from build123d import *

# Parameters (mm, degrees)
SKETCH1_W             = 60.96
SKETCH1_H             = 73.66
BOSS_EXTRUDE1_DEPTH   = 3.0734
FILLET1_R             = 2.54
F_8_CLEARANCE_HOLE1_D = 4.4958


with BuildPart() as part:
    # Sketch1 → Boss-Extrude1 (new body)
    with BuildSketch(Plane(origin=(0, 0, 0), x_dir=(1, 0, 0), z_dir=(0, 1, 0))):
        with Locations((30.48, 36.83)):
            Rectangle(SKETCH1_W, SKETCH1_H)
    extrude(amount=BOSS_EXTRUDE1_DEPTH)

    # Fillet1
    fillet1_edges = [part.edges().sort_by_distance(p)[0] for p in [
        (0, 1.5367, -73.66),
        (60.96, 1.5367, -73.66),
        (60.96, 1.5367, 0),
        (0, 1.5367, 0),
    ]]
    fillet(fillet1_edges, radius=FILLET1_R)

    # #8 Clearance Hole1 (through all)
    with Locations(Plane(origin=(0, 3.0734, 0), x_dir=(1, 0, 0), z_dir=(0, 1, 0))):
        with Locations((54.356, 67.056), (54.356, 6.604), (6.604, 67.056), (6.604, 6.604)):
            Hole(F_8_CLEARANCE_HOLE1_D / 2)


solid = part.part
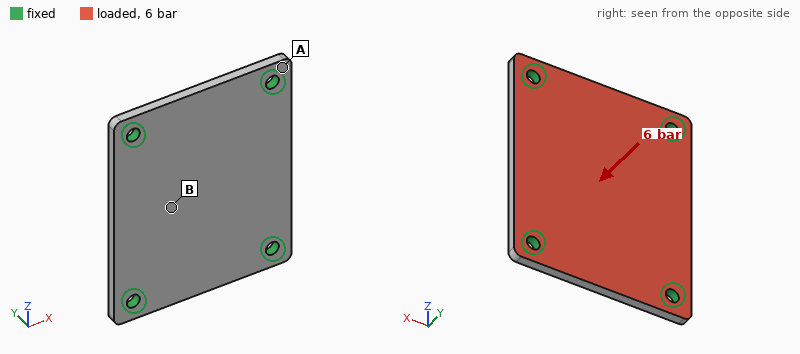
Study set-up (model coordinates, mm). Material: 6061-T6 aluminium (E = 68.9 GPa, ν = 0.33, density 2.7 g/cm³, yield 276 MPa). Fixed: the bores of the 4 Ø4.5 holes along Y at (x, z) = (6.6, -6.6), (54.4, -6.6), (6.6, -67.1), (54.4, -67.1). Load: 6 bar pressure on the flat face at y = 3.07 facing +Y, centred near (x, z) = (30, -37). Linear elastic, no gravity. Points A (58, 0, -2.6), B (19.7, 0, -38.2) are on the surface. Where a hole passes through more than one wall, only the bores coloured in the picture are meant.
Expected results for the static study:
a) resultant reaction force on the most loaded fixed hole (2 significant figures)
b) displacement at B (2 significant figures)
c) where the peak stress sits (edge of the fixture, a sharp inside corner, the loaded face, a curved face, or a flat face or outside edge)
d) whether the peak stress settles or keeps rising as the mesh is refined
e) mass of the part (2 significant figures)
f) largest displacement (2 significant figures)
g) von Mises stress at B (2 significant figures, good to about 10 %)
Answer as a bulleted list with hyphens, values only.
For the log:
- 660 N
- 0.18 mm
- edge of the fixture
- keeps rising
- 37 g
- 0.20 mm
- 58 MPa
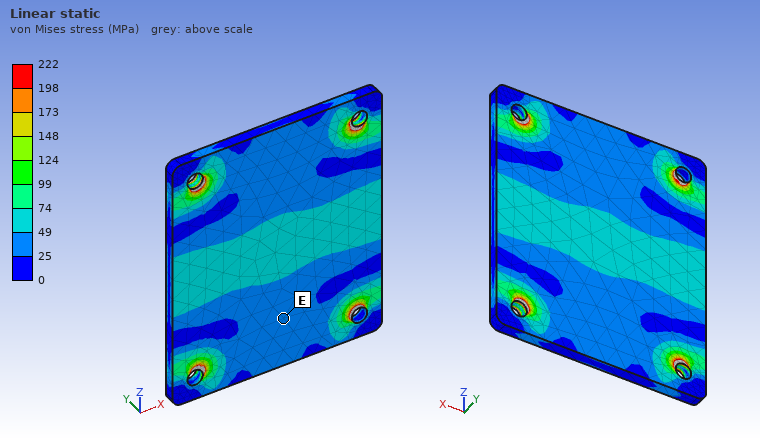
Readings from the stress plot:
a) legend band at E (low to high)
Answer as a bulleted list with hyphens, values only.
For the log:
- 25 to 49 MPa
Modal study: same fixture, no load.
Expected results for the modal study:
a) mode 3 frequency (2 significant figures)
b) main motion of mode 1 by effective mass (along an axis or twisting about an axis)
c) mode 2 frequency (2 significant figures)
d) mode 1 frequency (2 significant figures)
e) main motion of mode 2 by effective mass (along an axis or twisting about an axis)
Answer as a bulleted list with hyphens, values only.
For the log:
- 6900 Hz
- along Y
- 5400 Hz
- 3700 Hz
- twisting about Z
